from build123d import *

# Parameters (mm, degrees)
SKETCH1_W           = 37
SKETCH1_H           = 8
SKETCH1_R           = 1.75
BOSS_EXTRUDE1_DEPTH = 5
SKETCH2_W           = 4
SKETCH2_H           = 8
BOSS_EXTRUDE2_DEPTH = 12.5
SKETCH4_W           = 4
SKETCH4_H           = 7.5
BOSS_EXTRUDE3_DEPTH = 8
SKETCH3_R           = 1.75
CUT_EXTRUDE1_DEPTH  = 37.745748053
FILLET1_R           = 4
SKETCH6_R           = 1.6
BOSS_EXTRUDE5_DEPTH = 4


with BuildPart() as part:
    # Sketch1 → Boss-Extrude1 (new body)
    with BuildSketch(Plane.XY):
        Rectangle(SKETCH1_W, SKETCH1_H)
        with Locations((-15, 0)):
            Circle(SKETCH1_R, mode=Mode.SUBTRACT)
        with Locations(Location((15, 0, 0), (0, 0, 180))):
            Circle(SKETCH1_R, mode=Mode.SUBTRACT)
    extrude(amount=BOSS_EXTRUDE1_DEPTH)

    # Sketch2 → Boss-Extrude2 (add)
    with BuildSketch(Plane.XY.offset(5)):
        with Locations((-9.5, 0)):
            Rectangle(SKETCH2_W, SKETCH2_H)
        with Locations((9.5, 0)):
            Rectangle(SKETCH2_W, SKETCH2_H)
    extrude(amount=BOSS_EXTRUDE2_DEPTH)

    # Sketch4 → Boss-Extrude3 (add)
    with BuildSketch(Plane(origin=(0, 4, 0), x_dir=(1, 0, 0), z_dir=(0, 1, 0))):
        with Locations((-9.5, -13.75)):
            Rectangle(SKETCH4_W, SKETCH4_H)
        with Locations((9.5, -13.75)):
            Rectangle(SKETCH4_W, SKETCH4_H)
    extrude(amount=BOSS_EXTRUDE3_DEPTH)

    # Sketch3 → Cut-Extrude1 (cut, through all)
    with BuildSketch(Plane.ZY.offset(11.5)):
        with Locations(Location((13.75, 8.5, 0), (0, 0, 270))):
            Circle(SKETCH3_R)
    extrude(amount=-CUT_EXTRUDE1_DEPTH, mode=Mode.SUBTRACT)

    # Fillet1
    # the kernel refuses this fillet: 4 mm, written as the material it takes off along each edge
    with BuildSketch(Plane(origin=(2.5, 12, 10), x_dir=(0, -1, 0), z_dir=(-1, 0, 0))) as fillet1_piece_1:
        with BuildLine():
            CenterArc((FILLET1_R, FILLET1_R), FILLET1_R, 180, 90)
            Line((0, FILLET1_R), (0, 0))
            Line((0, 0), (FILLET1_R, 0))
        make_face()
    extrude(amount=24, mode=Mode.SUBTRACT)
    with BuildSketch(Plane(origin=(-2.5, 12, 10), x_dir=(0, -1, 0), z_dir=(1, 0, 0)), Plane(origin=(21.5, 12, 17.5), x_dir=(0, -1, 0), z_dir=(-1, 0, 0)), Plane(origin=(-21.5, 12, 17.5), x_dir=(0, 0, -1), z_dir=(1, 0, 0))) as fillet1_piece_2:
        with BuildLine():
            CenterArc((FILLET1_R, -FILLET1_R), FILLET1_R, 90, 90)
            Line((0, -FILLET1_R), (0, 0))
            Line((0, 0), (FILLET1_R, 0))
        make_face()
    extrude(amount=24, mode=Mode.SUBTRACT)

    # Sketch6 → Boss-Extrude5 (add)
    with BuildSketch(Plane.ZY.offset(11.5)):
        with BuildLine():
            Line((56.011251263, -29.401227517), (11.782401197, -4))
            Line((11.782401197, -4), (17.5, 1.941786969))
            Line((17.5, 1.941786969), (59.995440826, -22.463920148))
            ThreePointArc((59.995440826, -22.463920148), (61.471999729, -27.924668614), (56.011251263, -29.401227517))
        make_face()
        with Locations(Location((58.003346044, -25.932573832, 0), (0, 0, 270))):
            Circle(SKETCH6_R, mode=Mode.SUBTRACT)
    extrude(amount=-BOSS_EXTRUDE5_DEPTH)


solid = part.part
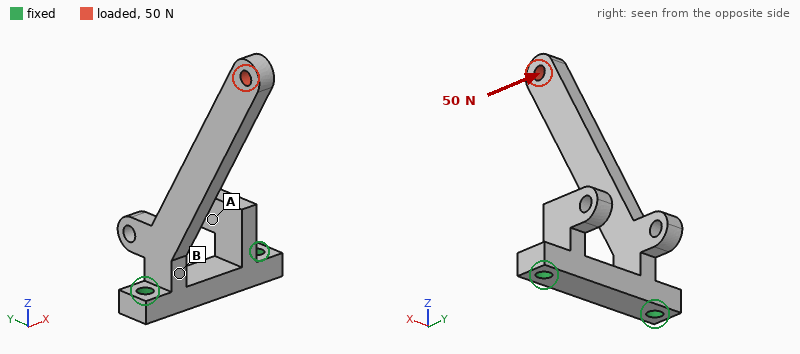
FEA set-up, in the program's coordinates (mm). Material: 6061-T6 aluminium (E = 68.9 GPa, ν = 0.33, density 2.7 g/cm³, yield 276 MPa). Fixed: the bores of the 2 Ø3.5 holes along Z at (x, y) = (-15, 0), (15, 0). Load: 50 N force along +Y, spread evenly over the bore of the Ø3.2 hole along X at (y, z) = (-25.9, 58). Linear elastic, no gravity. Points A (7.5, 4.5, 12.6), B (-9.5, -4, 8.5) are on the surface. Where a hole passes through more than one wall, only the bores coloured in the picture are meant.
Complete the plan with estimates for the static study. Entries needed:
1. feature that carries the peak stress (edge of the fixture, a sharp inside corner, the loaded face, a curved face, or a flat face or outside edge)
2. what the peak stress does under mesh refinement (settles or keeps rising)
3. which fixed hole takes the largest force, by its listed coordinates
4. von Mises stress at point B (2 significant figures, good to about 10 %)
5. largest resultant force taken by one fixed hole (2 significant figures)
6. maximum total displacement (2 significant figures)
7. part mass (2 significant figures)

edge of the fixture
keeps rising
(-15, 0)
55 MPa
54 N
0.40 mm
11 g
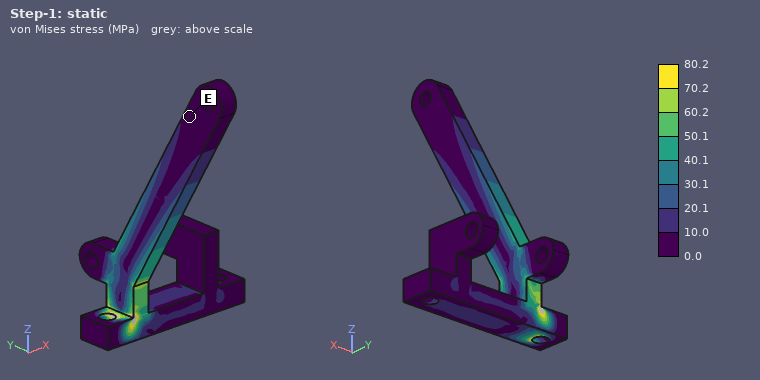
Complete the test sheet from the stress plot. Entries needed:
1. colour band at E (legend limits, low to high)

0.0 to 10.0 MPa
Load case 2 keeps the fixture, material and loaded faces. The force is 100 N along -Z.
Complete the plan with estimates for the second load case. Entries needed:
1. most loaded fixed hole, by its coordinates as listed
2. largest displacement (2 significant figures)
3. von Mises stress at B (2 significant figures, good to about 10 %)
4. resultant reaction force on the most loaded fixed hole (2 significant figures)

(-15, 0)
0.42 mm
61 MPa
91 N
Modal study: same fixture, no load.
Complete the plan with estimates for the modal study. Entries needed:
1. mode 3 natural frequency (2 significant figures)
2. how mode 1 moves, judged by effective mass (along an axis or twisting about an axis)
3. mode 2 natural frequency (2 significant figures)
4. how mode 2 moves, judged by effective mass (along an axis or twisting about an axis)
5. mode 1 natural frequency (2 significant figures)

4800 Hz
along X
1400 Hz
along Y
810 Hz
